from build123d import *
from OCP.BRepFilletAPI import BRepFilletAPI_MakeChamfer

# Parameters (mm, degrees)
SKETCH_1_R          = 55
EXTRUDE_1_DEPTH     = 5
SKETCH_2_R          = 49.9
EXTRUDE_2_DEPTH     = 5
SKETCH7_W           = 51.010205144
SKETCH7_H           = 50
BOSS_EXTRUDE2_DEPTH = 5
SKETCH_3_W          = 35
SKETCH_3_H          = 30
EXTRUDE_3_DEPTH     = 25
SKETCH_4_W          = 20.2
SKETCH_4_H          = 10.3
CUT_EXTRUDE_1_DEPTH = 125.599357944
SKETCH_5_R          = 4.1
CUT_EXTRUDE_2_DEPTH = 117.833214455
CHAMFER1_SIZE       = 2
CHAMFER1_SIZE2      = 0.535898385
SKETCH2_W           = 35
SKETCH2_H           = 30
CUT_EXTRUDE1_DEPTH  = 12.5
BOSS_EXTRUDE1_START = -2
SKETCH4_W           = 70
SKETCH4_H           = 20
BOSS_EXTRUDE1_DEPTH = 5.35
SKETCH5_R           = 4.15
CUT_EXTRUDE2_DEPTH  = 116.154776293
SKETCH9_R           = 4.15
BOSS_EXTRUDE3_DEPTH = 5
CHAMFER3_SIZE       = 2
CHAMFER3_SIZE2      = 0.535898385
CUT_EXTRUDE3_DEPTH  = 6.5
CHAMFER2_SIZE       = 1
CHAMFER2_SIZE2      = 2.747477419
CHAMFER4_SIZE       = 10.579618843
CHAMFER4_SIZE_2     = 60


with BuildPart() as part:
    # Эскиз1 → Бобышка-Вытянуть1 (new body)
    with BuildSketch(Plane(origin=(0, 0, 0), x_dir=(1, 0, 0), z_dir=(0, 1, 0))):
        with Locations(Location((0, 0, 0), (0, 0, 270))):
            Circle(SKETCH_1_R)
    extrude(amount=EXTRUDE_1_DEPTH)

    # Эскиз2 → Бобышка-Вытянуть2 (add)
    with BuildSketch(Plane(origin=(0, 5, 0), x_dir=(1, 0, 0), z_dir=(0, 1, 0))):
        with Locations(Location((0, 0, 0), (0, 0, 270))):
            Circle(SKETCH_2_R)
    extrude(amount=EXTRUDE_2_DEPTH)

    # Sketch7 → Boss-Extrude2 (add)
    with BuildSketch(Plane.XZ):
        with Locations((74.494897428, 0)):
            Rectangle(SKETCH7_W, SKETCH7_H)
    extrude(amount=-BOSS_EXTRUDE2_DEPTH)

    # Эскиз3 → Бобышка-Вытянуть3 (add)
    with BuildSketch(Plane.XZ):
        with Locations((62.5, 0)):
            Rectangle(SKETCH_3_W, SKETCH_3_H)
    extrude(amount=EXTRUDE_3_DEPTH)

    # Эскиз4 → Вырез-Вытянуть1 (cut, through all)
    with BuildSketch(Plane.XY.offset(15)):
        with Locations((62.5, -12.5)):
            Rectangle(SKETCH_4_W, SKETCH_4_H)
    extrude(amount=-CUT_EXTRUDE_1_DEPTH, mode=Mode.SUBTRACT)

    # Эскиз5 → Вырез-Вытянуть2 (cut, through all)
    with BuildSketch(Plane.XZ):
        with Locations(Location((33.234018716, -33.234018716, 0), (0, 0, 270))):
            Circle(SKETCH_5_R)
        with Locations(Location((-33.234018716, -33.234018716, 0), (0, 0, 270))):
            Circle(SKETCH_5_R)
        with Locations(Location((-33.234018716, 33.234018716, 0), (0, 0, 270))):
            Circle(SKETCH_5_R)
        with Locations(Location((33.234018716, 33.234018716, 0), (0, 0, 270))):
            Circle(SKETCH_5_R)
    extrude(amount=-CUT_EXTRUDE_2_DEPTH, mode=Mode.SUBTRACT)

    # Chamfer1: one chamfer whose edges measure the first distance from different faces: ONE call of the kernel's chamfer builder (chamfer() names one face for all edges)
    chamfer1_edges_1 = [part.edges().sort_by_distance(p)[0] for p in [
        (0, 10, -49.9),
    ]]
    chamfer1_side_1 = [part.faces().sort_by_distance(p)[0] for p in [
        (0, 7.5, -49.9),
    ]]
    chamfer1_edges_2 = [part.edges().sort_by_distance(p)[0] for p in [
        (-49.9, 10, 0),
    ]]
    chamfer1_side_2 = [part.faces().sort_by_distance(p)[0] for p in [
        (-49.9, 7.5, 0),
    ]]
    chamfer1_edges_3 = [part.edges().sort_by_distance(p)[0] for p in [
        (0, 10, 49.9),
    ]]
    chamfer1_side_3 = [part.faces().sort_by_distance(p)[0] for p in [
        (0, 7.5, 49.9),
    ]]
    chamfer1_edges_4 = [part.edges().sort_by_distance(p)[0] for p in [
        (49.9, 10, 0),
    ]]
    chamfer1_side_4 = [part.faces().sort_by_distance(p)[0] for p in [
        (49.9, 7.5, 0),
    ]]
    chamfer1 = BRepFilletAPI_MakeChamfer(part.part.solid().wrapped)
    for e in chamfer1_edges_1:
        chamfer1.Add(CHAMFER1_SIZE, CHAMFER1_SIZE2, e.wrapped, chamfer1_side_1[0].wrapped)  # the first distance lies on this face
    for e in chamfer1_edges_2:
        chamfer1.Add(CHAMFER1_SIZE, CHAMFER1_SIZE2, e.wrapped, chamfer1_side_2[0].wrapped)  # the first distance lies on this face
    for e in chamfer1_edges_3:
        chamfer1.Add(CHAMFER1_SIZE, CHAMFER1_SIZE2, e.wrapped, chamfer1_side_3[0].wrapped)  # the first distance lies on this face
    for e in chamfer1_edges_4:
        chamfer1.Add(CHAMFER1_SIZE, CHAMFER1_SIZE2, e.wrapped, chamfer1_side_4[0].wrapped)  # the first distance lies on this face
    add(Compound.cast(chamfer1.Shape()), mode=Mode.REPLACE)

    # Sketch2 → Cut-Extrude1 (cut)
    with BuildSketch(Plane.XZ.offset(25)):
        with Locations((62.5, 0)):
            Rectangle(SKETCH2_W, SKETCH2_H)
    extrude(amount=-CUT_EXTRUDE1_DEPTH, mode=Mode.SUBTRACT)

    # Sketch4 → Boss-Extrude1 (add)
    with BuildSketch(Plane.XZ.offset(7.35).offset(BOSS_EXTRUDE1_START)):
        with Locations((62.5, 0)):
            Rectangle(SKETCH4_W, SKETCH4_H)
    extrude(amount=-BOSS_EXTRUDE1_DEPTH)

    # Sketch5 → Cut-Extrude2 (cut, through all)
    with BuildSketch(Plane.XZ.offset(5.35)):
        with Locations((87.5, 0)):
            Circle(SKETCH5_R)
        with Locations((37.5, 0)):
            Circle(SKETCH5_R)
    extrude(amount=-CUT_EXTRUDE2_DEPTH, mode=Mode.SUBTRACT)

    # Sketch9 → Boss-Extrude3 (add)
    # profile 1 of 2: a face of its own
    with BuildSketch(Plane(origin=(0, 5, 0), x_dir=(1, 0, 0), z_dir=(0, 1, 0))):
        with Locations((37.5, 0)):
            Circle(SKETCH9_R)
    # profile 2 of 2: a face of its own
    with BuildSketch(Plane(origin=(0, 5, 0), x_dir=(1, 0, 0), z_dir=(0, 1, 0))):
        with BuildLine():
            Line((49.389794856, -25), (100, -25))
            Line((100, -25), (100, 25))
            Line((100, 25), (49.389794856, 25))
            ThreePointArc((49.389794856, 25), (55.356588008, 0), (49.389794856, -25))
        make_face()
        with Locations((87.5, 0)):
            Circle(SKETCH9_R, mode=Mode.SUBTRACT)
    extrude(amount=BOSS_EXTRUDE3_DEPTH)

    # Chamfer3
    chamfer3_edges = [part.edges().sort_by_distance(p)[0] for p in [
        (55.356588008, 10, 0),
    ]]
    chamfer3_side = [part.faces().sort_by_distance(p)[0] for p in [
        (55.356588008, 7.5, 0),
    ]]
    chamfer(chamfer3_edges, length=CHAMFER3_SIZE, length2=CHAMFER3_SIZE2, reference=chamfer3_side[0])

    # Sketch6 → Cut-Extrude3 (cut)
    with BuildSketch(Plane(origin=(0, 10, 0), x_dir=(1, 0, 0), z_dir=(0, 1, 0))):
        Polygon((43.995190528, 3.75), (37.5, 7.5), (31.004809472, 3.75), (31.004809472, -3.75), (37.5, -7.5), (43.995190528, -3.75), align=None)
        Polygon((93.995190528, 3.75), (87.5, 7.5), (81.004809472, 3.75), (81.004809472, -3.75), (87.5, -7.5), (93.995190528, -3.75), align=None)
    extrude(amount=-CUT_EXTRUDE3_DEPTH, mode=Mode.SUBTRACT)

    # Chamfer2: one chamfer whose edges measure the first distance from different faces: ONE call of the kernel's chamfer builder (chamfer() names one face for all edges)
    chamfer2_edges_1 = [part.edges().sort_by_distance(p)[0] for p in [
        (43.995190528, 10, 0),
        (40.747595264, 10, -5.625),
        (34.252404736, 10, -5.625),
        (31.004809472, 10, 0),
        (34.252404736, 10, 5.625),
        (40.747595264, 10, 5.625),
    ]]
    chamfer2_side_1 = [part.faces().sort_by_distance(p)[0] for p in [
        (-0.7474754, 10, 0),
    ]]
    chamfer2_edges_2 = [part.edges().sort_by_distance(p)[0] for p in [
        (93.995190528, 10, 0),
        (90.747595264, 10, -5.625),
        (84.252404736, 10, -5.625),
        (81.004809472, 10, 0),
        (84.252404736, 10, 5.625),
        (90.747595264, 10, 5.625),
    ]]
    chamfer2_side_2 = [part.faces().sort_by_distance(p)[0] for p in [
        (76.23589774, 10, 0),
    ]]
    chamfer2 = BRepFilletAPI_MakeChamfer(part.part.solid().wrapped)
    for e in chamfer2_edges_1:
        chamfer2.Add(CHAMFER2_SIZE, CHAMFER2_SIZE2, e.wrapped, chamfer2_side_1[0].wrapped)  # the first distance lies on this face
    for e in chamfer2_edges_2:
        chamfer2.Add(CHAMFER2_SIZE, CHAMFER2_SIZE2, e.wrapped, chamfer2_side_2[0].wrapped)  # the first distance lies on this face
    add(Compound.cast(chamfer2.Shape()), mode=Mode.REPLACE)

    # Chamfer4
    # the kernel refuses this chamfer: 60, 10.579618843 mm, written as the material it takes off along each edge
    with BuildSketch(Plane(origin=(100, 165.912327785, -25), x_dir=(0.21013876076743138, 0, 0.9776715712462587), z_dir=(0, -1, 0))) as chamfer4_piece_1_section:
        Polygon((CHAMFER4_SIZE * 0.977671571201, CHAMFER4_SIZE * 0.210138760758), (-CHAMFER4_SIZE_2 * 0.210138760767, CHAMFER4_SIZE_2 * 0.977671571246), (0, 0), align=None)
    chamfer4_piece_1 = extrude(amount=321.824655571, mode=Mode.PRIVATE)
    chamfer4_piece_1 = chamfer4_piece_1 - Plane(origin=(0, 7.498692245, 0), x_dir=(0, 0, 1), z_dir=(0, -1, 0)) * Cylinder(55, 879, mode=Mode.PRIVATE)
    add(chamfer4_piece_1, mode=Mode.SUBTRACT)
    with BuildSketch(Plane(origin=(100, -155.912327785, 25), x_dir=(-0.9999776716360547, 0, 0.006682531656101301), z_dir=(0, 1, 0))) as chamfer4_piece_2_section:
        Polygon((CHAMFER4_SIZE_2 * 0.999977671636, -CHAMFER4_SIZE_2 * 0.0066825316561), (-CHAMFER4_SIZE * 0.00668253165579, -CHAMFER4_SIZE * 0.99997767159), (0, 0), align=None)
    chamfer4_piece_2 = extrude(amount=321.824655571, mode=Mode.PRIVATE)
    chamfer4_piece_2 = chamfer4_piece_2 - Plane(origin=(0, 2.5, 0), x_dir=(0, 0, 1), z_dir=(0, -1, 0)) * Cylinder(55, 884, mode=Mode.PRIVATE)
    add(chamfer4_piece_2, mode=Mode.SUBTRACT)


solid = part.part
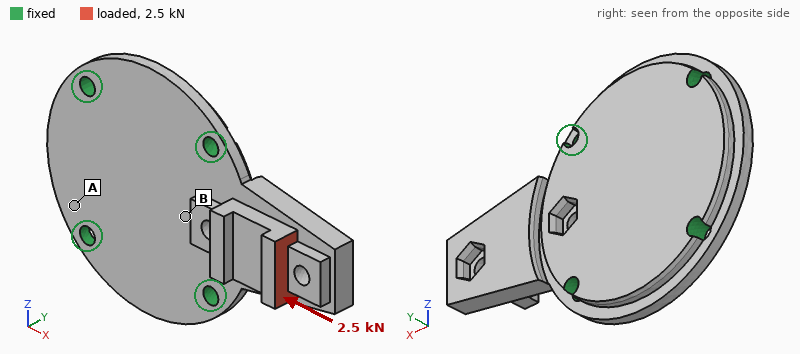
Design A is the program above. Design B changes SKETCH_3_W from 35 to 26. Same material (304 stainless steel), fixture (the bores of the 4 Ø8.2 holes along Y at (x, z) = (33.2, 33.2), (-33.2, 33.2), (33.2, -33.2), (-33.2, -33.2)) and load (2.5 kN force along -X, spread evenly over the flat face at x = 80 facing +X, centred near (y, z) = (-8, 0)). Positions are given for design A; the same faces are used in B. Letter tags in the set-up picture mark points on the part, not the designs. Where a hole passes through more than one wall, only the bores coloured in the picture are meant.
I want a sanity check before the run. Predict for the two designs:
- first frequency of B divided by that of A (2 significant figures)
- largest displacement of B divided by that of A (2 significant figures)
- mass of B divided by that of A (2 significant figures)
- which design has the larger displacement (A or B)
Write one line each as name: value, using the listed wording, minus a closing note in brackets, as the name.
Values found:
first frequency of B divided by that of A: 0.99
largest displacement of B divided by that of A: 1.1
mass of B divided by that of A: 0.98
which design has the larger displacement: B
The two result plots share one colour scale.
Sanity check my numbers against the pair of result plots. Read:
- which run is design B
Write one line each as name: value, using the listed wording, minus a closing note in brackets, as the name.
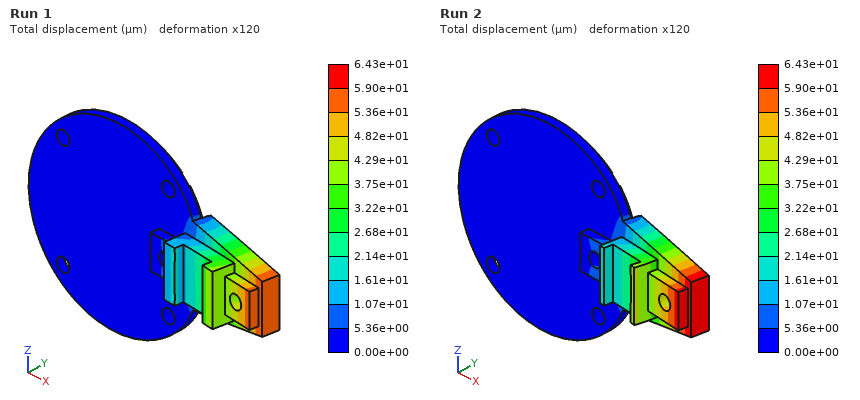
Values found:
which run is design B: Run 2
